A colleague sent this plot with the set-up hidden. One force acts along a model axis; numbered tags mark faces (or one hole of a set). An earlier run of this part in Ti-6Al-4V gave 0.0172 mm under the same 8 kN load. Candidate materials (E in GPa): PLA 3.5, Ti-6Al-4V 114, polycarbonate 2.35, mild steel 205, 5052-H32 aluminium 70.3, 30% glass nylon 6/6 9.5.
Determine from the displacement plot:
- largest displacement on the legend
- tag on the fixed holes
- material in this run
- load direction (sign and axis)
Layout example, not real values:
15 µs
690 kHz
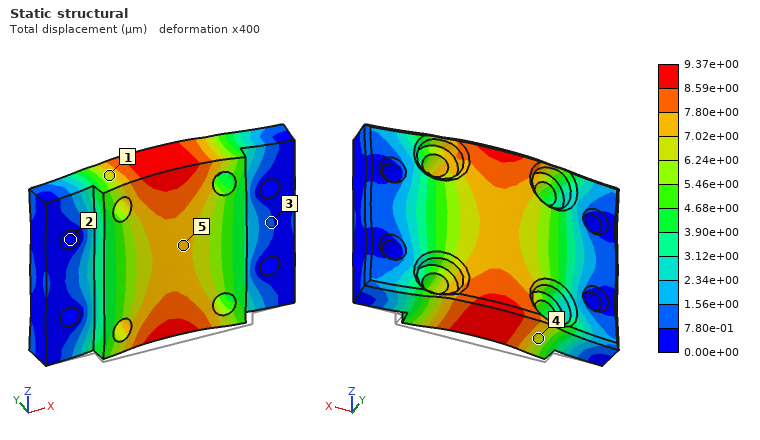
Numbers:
9.37e+00 µm
2
mild steel
+Y
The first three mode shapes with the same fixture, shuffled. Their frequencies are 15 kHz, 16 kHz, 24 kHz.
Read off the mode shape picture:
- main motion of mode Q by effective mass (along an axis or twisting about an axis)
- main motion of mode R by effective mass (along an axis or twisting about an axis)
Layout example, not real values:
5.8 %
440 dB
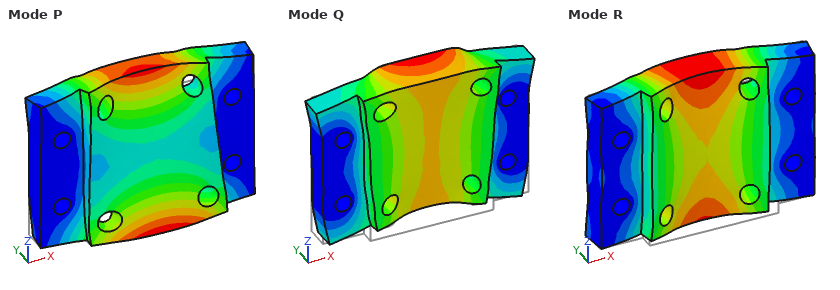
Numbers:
along Z
along Y
